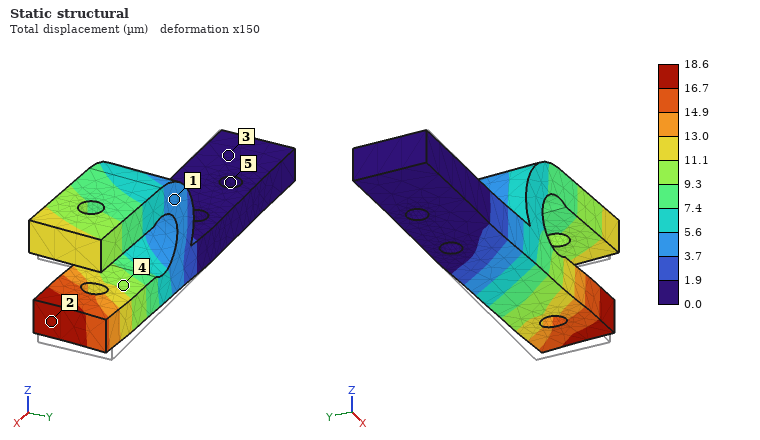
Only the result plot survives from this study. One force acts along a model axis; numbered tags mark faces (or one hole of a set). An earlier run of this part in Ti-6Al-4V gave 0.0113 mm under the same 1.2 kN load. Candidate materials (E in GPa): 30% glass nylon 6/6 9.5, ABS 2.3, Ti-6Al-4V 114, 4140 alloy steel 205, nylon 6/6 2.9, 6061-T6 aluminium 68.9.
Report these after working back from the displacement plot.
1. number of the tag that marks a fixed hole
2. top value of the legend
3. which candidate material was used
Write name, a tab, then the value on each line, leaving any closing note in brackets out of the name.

number of the tag that marks a fixed hole	5
top value of the legend	18.6 µm
which candidate material was used	6061-T6 aluminium
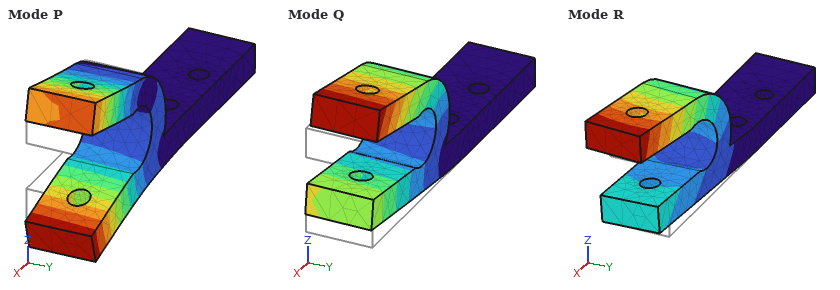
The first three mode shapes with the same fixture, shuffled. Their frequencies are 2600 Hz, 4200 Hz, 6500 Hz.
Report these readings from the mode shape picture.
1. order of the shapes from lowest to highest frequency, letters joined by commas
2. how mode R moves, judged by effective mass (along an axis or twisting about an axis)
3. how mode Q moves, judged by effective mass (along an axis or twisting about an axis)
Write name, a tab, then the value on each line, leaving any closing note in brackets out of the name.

order of the shapes from lowest to highest frequency, letters joined by commas	Q, R, P
how mode R moves, judged by effective mass	along Y
how mode Q moves, judged by effective mass	along Z
